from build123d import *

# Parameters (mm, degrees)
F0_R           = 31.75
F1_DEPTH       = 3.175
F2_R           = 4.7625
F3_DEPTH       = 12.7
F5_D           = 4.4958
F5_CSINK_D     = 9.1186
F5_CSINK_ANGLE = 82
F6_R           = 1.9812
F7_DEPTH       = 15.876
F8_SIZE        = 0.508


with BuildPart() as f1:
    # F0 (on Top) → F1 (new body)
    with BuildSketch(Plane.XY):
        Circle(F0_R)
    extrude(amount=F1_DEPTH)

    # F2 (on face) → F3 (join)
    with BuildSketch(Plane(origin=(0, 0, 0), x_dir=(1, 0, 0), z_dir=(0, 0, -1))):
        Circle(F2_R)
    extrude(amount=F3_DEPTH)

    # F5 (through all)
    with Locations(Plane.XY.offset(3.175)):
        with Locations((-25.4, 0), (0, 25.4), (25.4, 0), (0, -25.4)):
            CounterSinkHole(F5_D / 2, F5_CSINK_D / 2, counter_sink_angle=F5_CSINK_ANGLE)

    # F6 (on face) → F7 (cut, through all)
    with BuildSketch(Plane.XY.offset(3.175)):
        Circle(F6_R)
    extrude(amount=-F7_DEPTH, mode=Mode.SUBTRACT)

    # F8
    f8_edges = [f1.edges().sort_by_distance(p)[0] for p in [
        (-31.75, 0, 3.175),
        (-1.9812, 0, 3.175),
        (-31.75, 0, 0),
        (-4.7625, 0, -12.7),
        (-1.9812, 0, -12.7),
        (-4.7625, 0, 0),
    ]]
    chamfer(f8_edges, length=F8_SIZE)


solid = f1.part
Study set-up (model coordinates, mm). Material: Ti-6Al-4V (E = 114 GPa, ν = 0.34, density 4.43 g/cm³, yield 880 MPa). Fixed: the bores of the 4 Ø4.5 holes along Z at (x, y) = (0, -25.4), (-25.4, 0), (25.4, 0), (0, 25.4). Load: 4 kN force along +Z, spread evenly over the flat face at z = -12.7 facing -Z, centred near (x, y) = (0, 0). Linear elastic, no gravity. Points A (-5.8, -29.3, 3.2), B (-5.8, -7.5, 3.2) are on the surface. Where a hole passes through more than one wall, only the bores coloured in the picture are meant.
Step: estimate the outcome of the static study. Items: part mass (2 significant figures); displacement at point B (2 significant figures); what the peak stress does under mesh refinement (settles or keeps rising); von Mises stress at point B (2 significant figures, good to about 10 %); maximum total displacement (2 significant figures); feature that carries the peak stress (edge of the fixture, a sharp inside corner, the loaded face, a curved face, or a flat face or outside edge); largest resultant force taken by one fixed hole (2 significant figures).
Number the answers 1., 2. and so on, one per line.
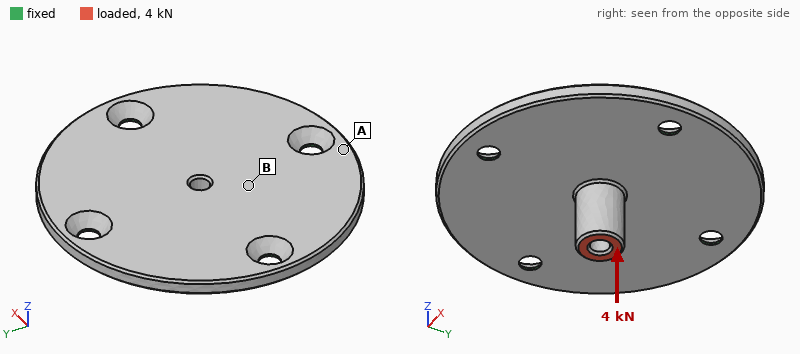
1. 46 g
2. 0.15 mm
3. keeps rising
4. 230 MPa
5. 0.20 mm
6. edge of the fixture
7. 2.6 kN
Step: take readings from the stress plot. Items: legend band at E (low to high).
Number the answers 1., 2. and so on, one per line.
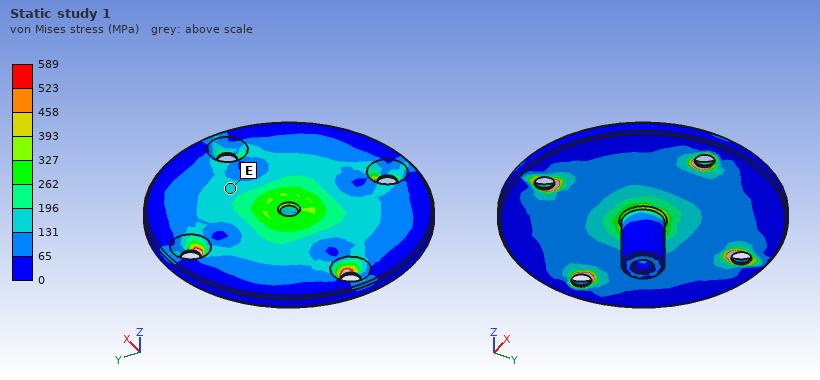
1. 131 to 196 MPa
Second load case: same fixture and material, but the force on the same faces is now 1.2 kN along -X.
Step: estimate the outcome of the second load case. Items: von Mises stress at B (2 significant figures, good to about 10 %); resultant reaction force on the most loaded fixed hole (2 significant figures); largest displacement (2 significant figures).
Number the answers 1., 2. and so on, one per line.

1. 81 MPa
2. 620 N
3. 0.11 mm
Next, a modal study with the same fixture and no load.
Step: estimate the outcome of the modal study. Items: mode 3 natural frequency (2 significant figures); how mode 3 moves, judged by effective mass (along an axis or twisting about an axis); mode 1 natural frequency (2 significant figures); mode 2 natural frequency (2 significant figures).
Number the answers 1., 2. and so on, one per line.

1. 7800 Hz
2. twisting about X
3. 6900 Hz
4. 7100 Hz
